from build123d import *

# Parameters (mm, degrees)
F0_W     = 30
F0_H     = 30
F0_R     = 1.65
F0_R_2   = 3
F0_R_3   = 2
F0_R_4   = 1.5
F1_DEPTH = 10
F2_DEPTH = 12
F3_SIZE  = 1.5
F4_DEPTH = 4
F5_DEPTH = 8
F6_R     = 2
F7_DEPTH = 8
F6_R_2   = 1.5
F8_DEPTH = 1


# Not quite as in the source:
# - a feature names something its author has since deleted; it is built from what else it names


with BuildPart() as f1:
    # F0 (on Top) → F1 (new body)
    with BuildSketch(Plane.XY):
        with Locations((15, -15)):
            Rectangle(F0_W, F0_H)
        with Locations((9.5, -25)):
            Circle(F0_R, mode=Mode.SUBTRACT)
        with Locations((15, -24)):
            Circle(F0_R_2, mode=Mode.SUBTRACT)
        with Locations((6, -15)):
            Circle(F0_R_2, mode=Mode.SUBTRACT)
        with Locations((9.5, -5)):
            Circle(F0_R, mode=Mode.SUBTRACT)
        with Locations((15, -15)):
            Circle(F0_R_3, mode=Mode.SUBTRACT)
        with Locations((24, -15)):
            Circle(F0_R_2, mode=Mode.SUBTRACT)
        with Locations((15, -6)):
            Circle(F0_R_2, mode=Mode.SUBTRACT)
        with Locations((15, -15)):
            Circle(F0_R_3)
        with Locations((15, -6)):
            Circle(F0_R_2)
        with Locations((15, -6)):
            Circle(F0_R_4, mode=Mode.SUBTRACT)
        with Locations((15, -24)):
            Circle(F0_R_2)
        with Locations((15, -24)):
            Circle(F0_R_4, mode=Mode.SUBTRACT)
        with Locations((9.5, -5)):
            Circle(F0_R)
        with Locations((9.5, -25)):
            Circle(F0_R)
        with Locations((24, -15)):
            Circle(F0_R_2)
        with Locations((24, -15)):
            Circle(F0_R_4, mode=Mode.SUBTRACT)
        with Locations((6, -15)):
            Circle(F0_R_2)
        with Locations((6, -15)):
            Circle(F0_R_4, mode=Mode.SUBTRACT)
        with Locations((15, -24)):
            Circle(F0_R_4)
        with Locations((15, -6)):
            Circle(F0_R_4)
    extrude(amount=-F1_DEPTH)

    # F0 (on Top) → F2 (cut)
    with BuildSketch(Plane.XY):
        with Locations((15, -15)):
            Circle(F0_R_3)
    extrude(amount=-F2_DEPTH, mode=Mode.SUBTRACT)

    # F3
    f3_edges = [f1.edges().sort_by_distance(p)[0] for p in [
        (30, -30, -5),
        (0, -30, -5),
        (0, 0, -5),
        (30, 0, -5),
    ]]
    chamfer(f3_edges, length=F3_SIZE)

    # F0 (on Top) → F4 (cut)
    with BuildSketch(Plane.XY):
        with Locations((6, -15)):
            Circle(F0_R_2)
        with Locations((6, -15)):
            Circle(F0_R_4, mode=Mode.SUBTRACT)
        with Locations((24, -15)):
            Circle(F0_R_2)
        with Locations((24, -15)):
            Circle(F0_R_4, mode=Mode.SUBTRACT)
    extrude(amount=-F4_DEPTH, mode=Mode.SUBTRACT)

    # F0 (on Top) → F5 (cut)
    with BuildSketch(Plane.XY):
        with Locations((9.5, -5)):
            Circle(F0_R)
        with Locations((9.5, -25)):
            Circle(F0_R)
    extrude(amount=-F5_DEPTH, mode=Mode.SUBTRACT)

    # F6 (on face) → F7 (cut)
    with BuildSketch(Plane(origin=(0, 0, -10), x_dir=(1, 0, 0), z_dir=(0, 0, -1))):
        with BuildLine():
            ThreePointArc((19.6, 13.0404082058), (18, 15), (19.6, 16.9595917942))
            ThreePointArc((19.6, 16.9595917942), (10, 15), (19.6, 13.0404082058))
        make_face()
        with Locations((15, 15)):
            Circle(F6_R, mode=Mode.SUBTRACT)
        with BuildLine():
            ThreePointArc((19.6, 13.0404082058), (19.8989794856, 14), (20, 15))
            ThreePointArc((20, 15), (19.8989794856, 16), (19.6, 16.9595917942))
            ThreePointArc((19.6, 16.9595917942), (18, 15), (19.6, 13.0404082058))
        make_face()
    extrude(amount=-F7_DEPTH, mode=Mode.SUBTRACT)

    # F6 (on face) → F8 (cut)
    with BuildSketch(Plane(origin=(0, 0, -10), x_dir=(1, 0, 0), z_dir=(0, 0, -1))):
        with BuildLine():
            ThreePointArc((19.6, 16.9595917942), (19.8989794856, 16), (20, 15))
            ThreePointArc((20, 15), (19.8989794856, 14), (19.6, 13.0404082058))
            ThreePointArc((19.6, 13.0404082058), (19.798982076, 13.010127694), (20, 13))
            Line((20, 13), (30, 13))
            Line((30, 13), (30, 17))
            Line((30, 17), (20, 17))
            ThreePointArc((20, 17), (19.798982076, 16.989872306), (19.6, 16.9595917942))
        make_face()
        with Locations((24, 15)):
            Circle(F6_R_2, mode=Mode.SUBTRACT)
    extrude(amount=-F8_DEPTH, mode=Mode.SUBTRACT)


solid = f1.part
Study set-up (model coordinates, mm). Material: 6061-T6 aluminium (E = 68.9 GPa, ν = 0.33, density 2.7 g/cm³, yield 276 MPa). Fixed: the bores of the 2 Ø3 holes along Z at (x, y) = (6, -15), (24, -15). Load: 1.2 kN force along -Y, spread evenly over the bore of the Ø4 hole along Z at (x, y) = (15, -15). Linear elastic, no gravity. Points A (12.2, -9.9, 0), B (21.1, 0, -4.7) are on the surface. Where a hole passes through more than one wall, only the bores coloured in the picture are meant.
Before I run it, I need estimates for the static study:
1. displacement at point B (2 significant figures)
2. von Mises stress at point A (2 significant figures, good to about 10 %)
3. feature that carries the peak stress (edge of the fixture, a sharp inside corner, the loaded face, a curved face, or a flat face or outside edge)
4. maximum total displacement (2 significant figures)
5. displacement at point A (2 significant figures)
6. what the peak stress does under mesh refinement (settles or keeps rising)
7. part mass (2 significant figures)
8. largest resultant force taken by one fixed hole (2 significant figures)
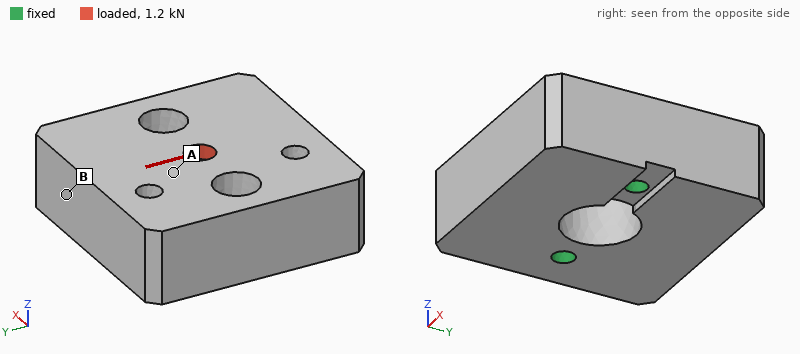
11 µm
21 MPa
edge of the fixture
12 µm
7.2 µm
keeps rising
21 g
600 N
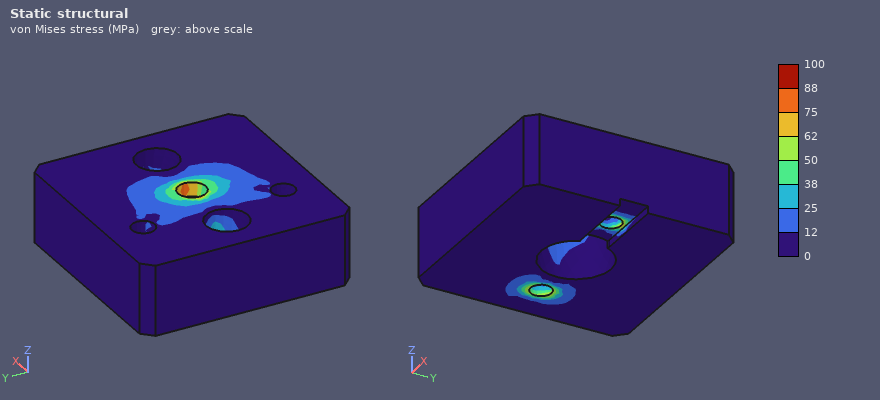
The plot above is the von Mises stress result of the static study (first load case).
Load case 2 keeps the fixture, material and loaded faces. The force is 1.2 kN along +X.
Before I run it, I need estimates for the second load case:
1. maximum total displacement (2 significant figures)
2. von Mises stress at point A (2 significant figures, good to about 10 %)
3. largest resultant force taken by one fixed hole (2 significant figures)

6.3 µm
10 MPa
670 N
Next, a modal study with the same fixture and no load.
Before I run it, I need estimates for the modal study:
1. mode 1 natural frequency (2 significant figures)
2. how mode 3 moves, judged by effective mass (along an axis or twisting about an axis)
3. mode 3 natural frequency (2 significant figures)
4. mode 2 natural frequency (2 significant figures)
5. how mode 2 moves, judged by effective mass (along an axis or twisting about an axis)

12 kHz
twisting about Z
25 kHz
22 kHz
along Z
